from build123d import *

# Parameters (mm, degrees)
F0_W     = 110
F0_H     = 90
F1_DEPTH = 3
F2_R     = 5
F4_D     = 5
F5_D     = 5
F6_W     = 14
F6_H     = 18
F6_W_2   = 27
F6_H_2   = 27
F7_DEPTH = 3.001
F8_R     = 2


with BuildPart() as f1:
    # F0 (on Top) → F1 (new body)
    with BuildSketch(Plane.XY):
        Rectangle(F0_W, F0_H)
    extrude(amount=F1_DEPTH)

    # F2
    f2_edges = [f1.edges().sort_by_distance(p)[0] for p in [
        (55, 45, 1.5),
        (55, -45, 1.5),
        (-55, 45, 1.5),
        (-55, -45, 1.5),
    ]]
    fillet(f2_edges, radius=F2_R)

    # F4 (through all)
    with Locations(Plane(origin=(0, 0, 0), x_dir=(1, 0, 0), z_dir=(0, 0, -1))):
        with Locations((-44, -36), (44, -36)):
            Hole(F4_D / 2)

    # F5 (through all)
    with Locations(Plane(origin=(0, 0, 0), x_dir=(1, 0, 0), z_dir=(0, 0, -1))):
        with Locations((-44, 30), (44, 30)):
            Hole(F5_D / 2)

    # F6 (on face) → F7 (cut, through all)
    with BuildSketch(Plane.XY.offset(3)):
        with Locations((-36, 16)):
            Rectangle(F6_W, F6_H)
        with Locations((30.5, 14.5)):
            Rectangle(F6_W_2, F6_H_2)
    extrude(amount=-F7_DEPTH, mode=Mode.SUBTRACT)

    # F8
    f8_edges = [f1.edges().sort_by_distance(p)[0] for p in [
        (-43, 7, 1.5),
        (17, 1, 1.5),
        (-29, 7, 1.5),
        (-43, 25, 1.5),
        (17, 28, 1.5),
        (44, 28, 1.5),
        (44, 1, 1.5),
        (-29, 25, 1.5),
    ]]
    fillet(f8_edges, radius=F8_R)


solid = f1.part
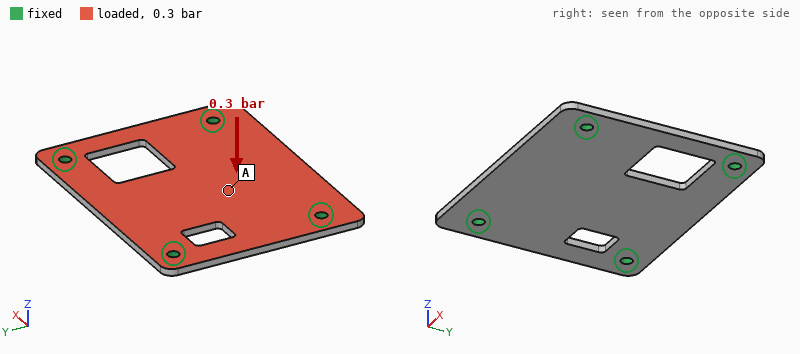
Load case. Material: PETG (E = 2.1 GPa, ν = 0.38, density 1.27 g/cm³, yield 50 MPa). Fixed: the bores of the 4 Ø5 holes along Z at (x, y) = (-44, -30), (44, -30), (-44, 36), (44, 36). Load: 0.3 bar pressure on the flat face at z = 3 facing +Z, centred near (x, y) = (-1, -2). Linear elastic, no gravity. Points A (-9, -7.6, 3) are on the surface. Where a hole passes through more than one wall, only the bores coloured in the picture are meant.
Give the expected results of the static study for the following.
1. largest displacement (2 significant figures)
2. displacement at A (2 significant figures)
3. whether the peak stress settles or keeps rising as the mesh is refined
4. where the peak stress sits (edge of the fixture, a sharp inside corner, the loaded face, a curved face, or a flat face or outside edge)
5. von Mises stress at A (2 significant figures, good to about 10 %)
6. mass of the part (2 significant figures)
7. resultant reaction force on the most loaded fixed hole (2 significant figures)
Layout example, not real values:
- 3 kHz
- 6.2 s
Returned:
- 1.5 mm
- 1.3 mm
- keeps rising
- edge of the fixture
- 5.5 MPa
- 34 g
- 77 N
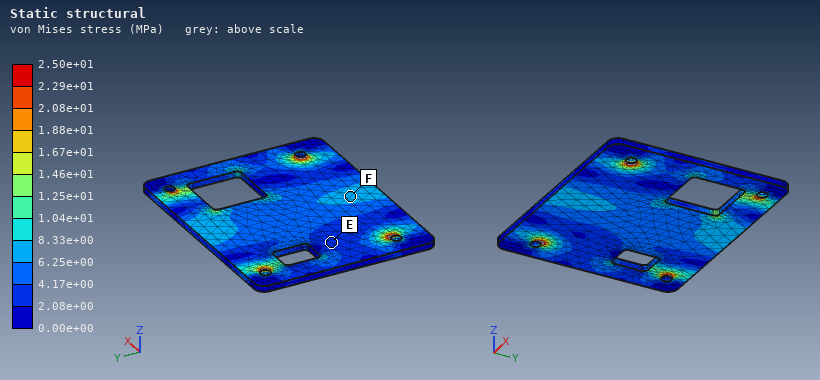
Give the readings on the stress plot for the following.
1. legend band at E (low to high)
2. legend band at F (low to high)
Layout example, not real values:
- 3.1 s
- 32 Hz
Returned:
- 2.08e+00 to 4.17e+00 MPa
- 6.25e+00 to 8.33e+00 MPa
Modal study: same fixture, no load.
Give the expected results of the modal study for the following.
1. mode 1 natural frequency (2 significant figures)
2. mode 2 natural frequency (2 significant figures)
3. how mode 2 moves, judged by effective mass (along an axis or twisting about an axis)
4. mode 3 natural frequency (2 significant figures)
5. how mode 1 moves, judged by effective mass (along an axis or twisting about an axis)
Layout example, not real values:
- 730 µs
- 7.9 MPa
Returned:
- 430 Hz
- 590 Hz
- twisting about X
- 790 Hz
- along Z
